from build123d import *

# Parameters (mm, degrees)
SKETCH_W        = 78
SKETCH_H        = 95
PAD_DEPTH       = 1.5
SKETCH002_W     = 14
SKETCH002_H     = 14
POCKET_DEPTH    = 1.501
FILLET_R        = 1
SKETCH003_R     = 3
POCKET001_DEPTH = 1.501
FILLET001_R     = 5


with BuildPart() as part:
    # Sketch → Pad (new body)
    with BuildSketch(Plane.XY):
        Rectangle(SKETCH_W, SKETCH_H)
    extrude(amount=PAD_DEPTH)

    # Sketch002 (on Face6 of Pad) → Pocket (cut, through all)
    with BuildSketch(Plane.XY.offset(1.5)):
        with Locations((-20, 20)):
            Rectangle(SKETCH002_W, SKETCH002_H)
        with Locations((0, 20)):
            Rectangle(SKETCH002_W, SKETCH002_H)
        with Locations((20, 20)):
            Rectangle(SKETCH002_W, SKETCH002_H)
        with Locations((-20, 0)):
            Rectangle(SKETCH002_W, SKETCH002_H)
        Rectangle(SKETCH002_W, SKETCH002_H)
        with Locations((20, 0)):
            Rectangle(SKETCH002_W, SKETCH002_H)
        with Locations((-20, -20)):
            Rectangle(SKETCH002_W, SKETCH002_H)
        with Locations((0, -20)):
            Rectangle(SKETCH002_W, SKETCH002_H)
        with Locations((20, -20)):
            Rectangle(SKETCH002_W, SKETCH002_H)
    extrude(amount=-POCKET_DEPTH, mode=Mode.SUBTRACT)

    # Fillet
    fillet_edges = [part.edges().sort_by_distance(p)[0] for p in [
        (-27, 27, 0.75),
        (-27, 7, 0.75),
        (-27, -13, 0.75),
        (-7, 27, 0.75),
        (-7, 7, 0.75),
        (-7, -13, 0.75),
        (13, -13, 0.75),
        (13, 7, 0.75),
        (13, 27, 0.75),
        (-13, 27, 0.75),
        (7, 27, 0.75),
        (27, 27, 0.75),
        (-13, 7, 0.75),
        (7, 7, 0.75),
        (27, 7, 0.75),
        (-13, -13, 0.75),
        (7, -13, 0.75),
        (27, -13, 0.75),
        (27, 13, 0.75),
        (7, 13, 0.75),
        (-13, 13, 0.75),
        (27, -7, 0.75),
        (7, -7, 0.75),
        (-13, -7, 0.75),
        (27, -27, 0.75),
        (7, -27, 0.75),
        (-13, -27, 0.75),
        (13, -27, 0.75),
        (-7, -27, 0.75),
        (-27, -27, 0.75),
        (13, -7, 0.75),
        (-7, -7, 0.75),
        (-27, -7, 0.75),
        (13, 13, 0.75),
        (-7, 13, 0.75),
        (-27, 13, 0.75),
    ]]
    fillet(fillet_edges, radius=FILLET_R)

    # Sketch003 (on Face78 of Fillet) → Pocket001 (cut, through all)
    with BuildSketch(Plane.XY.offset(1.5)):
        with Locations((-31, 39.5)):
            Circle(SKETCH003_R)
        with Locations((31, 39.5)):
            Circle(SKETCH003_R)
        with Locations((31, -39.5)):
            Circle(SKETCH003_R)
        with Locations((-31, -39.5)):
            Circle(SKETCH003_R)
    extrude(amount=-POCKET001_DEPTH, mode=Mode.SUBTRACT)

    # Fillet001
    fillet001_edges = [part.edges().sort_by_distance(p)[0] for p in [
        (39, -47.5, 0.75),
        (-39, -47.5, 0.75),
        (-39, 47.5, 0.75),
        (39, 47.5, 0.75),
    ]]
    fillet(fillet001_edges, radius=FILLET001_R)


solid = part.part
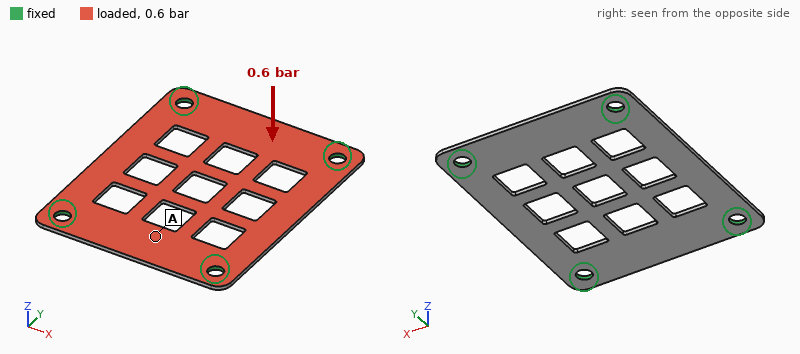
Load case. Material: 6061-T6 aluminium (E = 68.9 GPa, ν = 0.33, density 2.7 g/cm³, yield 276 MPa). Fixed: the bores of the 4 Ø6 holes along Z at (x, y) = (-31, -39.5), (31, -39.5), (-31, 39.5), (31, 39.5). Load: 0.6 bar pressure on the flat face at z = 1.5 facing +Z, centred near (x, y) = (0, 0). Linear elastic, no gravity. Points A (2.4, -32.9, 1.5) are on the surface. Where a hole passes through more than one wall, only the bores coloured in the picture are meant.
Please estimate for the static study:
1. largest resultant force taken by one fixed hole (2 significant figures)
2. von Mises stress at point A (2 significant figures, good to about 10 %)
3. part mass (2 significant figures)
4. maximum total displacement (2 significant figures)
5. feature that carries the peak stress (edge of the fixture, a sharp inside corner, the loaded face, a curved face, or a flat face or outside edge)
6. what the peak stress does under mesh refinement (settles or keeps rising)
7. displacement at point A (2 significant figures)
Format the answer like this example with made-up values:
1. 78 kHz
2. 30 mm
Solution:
1. 83 N
2. 32 MPa
3. 22 g
4. 0.43 mm
5. edge of the fixture
6. keeps rising
7. 0.17 mm
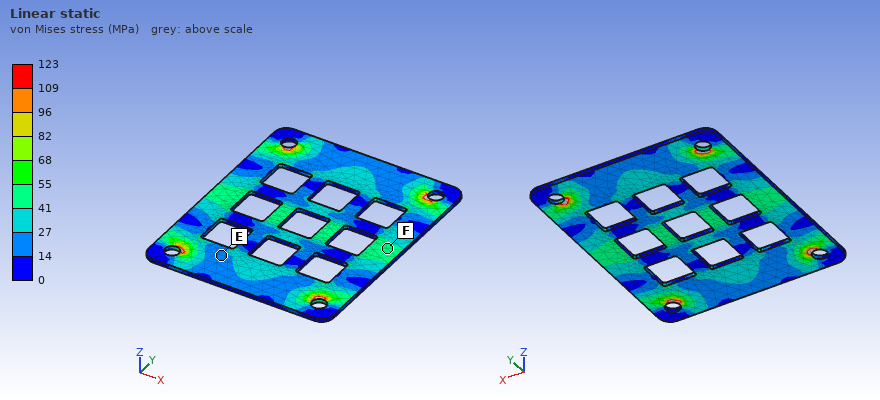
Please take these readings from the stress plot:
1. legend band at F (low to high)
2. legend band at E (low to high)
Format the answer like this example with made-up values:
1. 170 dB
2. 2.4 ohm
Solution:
1. 41 to 55 MPa
2. 14 to 27 MPa
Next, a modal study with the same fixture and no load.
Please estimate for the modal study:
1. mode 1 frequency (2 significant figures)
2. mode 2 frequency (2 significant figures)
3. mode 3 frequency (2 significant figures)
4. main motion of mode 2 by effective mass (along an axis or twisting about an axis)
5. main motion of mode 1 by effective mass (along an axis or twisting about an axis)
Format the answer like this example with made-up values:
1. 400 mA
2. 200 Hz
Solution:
1. 1200 Hz
2. 1600 Hz
3. 1900 Hz
4. twisting about Y
5. along Z
